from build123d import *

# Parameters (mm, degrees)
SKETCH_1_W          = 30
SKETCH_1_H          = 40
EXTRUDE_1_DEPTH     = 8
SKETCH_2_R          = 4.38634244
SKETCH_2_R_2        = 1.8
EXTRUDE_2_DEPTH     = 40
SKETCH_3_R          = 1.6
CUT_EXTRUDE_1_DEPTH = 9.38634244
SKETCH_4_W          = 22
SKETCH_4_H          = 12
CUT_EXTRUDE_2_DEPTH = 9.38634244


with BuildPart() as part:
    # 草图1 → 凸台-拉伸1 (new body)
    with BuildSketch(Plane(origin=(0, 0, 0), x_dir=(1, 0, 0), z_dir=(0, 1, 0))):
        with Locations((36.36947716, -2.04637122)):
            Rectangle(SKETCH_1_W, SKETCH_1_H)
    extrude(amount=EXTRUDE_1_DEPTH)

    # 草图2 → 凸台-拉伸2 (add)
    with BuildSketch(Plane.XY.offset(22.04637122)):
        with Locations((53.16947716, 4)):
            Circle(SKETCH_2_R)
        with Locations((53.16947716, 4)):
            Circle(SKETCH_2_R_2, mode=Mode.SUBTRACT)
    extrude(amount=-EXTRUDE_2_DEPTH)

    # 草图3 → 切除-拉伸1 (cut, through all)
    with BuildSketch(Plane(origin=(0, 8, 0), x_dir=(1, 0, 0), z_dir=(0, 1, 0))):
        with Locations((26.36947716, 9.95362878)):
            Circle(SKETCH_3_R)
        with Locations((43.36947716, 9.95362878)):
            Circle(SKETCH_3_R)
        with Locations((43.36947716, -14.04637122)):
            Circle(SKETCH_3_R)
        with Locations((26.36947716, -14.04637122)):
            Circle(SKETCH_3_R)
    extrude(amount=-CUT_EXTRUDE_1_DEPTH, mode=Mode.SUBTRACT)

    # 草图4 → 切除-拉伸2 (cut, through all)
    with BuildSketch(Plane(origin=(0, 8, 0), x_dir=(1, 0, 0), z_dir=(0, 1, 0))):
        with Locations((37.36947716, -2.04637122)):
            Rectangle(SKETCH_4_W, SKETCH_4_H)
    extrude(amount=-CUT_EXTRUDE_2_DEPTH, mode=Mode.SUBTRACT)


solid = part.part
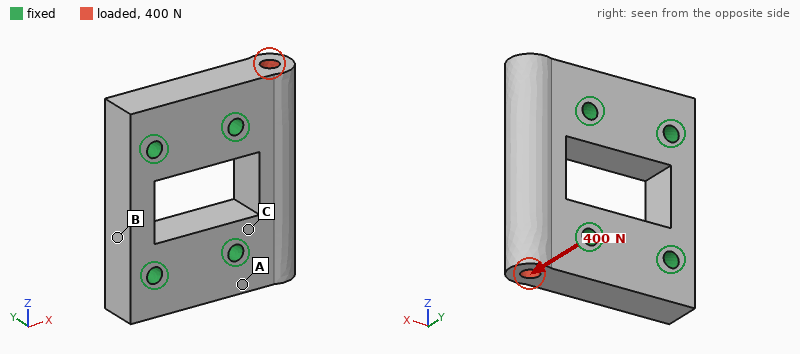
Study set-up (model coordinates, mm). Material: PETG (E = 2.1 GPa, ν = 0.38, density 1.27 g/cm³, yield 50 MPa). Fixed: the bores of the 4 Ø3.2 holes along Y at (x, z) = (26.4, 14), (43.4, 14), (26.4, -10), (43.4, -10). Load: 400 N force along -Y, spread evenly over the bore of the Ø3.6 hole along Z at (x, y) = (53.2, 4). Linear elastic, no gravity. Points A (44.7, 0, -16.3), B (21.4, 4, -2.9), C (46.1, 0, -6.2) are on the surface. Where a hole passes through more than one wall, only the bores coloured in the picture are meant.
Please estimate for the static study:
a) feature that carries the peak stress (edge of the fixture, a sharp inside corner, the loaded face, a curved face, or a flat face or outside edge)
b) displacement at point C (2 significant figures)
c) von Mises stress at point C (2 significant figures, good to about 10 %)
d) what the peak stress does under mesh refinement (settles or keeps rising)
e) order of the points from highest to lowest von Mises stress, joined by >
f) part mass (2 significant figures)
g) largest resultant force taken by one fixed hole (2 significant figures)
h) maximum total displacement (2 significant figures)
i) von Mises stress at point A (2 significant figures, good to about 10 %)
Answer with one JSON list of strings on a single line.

["edge of the fixture", "0.031 mm", "8.5 MPa", "keeps rising", "C > A > B", "11 g", "230 N", "0.15 mm", "5.5 MPa"]
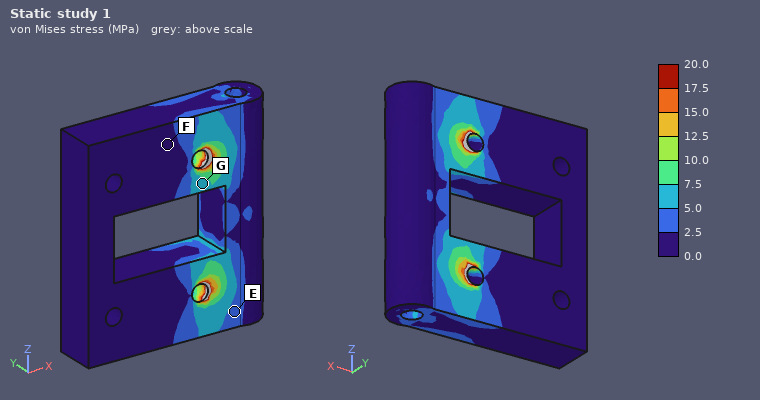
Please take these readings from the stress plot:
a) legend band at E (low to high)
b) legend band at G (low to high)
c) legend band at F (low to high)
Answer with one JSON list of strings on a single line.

["2.5 to 5.0 MPa", "5.0 to 7.5 MPa", "0.0 to 2.5 MPa"]
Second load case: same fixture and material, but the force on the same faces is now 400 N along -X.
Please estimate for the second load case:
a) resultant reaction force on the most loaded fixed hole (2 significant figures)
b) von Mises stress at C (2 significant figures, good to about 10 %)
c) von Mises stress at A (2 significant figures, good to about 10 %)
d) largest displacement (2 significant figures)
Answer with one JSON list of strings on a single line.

["180 N", "2.3 MPa", "0.77 MPa", "23 µm"]
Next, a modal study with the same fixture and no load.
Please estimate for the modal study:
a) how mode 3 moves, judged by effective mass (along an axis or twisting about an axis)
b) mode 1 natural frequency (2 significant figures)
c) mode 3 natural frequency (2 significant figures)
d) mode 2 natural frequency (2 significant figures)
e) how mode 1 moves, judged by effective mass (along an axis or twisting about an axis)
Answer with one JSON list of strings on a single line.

["along Z", "5900 Hz", "9000 Hz", "7900 Hz", "along Y"]
